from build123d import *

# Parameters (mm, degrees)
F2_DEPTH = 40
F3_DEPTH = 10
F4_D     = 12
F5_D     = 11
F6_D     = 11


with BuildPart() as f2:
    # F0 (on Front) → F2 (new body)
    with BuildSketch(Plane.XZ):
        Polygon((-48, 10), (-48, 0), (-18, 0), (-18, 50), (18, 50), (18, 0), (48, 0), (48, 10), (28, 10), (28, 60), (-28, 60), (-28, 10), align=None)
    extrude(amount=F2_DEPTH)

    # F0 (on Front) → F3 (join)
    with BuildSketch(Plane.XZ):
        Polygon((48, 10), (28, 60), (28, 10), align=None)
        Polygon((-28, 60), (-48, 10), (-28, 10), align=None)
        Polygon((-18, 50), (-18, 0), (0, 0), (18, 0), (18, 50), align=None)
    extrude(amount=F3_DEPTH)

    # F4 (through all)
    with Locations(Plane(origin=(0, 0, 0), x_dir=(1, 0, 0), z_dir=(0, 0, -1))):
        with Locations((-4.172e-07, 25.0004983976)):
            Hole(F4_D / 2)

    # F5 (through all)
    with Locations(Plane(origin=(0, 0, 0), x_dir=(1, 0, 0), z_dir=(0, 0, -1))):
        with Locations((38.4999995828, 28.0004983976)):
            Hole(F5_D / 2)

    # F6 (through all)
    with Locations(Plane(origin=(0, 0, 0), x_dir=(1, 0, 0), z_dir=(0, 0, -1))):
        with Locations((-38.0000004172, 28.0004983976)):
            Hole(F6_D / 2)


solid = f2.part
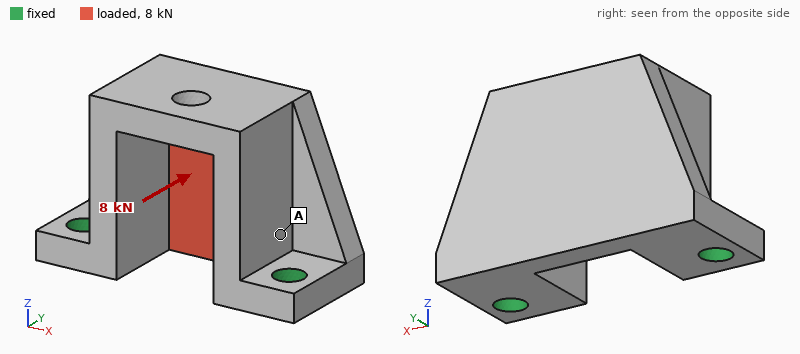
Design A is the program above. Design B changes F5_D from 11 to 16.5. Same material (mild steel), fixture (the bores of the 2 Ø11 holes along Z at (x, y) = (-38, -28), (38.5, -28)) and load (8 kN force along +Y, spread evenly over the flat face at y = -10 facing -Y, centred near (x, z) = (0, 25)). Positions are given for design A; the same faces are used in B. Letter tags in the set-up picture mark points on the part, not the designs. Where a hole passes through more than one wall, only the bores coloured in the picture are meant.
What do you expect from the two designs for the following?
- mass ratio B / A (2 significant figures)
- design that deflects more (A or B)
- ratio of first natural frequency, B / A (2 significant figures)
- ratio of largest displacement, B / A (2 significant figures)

0.99
A
1.1
0.81
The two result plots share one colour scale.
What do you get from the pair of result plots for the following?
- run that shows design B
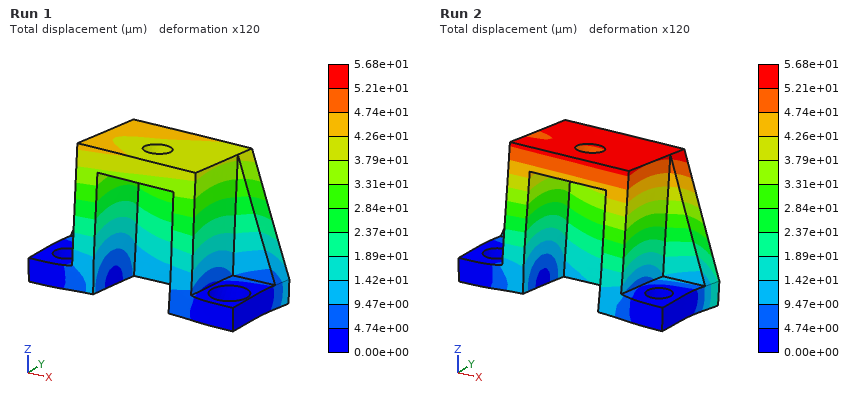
Run 1
